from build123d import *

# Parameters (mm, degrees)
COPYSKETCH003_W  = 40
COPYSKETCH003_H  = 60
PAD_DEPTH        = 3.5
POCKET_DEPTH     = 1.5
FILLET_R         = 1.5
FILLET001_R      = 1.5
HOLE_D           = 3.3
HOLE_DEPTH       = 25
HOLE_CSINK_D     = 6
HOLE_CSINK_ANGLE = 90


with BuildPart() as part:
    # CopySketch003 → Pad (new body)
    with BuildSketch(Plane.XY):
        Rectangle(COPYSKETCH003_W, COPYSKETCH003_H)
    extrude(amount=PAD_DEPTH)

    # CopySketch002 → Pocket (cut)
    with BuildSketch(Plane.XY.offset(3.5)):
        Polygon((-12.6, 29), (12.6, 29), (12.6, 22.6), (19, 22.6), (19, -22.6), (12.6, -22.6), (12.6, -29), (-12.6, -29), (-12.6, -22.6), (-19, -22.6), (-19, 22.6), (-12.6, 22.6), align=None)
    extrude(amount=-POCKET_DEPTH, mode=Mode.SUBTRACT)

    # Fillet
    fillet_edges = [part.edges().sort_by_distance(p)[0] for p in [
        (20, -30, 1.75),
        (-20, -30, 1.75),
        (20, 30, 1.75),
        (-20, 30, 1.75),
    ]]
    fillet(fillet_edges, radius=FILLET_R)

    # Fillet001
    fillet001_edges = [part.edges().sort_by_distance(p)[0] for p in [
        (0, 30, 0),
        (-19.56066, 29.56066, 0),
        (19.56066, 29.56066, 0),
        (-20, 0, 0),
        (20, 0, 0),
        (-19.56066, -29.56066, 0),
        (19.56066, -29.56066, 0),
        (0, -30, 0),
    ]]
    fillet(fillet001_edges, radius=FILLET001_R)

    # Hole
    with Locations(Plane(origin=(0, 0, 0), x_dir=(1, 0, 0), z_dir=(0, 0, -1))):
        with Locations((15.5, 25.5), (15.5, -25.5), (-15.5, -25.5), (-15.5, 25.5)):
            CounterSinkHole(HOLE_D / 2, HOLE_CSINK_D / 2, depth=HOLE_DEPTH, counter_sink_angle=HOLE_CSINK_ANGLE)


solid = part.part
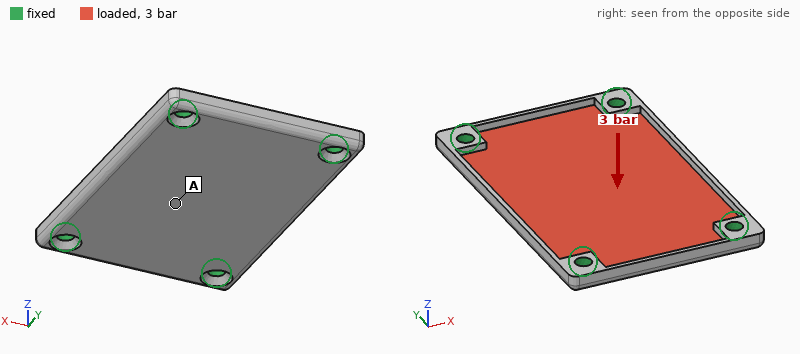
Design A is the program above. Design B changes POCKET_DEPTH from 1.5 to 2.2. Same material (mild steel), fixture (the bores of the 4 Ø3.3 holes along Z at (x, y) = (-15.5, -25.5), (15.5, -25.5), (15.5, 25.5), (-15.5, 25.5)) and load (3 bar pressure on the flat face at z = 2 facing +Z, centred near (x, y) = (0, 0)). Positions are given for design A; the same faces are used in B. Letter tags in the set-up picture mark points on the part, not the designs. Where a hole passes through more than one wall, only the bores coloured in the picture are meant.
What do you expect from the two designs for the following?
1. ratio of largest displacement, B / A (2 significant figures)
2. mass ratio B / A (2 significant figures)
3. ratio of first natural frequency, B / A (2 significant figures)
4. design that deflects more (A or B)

2.6
0.72
0.81
B
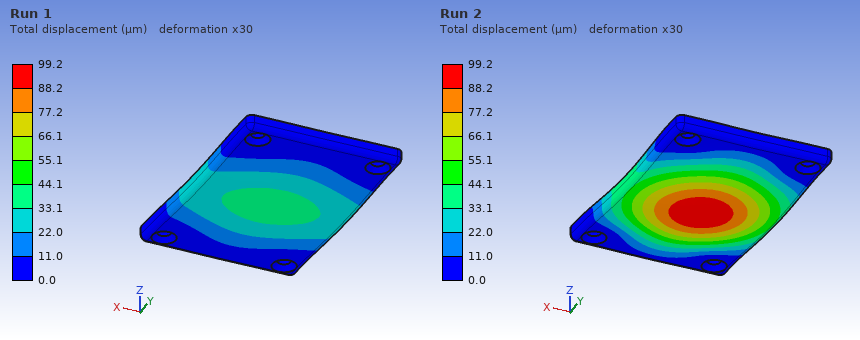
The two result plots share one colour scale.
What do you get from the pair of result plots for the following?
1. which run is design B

Run 2
